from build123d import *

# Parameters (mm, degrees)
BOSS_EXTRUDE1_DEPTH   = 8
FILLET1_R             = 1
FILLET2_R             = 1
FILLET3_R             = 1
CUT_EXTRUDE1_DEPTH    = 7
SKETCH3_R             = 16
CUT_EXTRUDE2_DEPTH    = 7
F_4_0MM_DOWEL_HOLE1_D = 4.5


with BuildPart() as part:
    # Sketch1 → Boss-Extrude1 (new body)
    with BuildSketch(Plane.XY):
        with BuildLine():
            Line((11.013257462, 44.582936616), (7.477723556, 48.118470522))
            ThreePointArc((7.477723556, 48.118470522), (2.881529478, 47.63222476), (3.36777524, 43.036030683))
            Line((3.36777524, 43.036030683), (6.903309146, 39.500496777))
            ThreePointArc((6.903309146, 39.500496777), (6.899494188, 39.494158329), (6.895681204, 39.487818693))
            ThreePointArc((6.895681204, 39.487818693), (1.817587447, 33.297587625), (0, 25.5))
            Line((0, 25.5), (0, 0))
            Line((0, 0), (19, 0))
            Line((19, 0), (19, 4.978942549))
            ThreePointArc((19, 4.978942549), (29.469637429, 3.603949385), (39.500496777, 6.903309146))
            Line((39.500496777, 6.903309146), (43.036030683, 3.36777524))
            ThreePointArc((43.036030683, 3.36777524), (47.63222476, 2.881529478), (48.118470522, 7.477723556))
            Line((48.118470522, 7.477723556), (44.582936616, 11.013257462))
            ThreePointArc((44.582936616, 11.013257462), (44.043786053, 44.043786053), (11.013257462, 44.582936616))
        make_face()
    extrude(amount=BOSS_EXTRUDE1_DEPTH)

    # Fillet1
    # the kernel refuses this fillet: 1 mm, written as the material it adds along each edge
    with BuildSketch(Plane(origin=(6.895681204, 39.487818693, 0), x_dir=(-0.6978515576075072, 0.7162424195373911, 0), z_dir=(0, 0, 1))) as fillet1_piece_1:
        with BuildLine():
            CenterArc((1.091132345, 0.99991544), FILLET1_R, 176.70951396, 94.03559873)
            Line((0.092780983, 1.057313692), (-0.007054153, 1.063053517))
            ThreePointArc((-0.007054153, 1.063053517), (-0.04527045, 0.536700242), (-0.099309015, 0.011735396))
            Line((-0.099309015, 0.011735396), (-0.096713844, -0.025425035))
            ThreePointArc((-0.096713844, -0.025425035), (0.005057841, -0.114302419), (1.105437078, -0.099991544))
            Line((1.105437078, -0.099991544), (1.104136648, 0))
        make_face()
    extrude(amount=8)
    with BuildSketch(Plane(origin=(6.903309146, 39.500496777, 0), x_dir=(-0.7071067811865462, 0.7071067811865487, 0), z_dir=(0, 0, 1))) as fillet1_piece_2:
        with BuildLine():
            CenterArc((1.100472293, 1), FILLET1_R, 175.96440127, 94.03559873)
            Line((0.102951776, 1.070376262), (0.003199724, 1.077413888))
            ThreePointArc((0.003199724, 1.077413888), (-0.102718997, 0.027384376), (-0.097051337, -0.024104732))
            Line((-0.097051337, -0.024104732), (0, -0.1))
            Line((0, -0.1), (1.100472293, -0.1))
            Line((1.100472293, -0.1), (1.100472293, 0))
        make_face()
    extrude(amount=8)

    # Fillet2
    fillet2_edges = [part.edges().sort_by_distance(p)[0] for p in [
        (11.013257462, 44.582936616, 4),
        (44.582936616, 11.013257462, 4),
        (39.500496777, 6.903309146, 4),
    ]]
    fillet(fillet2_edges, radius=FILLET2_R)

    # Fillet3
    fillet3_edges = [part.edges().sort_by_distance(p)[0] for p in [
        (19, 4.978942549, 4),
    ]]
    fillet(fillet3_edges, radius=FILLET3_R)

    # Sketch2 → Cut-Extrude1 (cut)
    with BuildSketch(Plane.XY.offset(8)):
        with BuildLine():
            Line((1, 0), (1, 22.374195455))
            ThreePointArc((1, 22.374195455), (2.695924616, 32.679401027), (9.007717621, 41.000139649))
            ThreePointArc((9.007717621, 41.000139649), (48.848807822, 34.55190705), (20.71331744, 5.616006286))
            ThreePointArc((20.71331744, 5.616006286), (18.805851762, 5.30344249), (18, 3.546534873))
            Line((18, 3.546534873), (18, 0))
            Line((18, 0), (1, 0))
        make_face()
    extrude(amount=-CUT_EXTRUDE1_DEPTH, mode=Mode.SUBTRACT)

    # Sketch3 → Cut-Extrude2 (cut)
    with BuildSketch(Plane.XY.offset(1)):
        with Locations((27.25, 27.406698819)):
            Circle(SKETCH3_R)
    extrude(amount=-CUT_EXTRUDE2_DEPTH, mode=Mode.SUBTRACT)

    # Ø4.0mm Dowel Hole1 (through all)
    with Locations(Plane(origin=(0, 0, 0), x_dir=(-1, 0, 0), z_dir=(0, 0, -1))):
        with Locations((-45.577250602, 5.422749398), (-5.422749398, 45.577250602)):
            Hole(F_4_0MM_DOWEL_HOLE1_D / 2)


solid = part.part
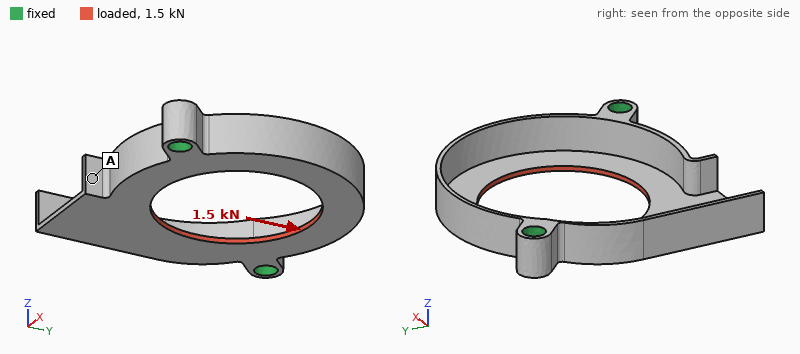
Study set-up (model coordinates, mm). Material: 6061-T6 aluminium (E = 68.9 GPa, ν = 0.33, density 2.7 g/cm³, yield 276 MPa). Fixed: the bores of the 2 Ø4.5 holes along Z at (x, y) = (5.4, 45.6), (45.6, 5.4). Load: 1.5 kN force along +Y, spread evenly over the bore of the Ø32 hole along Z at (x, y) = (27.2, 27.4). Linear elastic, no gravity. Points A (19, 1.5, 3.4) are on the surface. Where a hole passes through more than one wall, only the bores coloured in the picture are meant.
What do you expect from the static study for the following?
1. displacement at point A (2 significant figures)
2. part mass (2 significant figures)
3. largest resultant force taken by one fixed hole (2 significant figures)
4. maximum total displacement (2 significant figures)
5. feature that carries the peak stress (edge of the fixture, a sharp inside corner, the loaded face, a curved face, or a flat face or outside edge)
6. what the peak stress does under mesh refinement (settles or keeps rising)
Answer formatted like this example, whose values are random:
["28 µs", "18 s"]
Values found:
["33 µm", "7.6 g", "770 N", "91 µm", "a sharp inside corner", "keeps rising"]
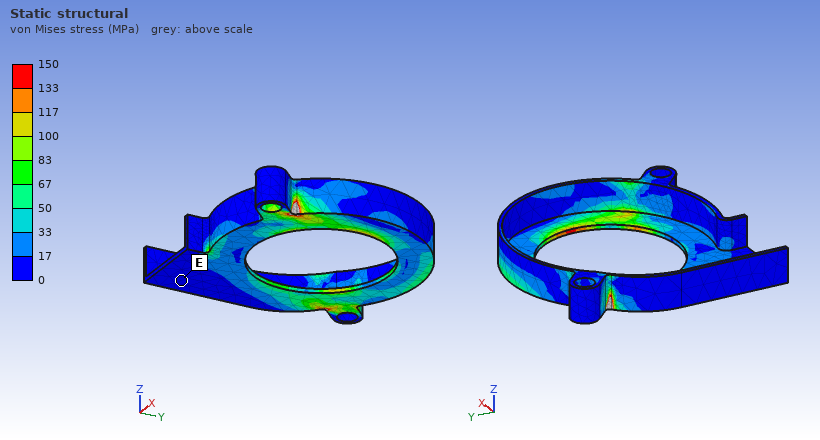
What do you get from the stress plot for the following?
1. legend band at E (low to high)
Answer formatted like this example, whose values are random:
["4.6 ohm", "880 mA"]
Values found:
["0 to 17 MPa"]
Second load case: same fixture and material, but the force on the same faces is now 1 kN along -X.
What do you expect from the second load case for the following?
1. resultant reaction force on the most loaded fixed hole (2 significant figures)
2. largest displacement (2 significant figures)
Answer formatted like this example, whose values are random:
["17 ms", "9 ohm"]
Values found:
["520 N", "63 µm"]
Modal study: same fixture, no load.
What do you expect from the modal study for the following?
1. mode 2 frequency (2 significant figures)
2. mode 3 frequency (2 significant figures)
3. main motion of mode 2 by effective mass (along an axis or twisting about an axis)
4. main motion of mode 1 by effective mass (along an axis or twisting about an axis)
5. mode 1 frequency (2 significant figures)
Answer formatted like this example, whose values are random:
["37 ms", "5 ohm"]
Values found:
["3700 Hz", "4500 Hz", "along Z", "along Z", "2200 Hz"]
